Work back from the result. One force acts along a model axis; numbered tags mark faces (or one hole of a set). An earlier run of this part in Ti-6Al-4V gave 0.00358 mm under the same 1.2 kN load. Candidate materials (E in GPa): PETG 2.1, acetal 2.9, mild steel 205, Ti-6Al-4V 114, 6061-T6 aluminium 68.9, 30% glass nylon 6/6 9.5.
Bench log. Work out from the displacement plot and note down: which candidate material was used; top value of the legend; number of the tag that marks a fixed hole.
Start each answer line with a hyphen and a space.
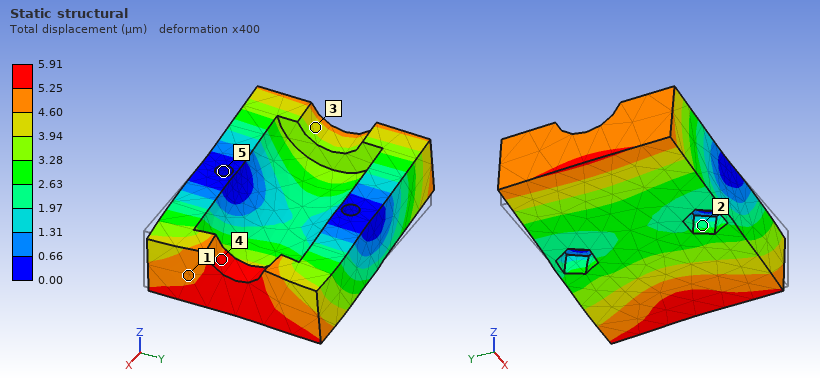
- 6061-T6 aluminium
- 5.91 µm
- 5
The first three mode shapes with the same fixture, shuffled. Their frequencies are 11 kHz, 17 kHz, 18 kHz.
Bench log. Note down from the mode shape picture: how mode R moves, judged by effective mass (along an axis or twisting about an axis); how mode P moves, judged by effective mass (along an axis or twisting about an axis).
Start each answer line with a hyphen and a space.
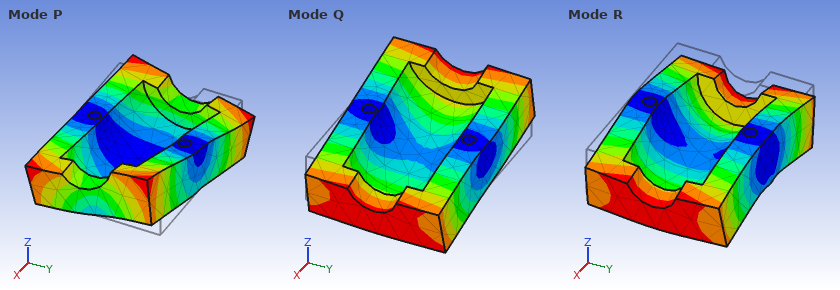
- along Z
- twisting about Z
